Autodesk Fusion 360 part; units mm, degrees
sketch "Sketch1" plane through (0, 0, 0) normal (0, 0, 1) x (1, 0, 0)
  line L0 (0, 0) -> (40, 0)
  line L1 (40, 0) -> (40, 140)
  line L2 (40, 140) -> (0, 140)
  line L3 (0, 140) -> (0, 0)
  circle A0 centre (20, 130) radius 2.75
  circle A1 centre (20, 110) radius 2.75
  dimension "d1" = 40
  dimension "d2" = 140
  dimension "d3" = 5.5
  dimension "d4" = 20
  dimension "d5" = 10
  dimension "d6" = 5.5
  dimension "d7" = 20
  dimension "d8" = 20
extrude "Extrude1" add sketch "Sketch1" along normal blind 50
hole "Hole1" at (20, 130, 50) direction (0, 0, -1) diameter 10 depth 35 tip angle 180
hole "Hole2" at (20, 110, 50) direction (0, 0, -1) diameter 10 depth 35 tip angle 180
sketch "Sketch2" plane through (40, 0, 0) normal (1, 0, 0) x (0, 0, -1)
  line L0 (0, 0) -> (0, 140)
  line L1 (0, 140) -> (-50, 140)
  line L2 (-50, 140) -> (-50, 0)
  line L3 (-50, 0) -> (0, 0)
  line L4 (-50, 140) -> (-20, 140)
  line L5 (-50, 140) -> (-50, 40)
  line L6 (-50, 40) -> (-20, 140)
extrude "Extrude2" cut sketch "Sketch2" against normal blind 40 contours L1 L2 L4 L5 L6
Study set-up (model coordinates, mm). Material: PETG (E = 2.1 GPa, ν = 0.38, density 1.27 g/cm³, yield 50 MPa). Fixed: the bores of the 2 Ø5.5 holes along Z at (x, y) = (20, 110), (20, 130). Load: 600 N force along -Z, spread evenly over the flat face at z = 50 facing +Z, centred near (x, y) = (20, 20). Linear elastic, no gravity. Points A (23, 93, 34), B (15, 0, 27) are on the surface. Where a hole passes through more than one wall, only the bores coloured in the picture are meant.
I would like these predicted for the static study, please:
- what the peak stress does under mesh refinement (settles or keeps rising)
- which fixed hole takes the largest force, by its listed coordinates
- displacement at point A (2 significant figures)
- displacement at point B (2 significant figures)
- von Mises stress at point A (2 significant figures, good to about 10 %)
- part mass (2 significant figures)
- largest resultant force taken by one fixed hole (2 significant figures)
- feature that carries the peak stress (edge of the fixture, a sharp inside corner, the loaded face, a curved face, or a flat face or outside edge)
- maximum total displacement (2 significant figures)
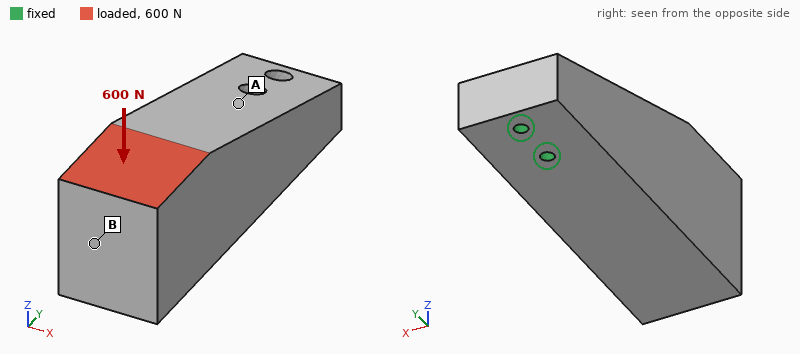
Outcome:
keeps rising
(20, 110)
0.36 mm
1.6 mm
4.4 MPa
280 g
2.2 kN
edge of the fixture
1.7 mm
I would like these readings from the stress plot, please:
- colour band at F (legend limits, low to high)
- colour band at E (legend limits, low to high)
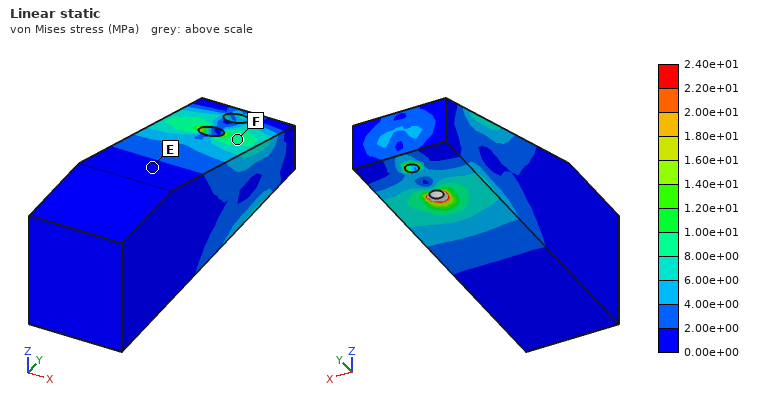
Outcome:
8.00e+00 to 1.00e+01 MPa
0.00e+00 to 2.00e+00 MPa
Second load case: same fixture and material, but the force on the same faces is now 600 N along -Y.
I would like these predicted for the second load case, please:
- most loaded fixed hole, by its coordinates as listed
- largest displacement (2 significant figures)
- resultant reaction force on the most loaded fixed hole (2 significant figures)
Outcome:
(20, 130)
0.80 mm
860 N
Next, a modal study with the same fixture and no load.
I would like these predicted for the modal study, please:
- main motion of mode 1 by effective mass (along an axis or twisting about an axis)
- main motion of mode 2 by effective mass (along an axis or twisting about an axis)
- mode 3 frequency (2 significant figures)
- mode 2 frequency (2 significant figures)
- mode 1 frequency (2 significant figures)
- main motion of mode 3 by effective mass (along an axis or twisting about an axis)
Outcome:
along Z
along X
860 Hz
320 Hz
290 Hz
twisting about Y
